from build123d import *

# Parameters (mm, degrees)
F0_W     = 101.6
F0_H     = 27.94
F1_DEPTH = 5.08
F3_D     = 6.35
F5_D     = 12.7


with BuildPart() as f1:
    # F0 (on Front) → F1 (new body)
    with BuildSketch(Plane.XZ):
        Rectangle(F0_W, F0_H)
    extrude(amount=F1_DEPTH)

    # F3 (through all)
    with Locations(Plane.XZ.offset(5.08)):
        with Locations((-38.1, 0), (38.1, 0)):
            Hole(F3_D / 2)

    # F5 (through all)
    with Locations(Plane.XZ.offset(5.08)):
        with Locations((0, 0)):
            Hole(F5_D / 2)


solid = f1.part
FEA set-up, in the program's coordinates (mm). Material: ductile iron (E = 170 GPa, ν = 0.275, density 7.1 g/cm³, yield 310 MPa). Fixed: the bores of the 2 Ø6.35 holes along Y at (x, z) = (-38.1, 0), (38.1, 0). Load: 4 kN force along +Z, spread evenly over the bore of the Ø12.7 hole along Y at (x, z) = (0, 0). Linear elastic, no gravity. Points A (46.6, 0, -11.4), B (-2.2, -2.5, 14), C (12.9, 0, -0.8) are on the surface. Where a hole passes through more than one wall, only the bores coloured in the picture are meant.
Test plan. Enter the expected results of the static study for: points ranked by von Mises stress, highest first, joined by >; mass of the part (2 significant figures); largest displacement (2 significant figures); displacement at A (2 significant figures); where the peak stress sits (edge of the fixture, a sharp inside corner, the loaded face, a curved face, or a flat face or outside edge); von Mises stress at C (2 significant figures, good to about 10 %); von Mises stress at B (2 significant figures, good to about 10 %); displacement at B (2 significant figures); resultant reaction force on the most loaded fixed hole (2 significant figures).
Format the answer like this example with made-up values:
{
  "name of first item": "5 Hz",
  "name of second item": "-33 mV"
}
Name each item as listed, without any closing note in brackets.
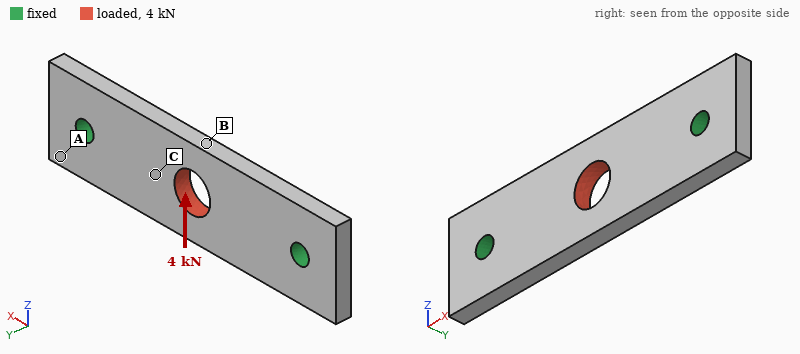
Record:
{
  "points ranked by von Mises stress, highest first, joined by >": "B > C > A",
  "mass of the part": "96 g",
  "largest displacement": "22 µm",
  "displacement at A": "5.6 µm",
  "where the peak stress sits": "edge of the fixture",
  "von Mises stress at C": "34 MPa",
  "von Mises stress at B": "85 MPa",
  "displacement at B": "21 µm",
  "resultant reaction force on the most loaded fixed hole": "2.0 kN"
}
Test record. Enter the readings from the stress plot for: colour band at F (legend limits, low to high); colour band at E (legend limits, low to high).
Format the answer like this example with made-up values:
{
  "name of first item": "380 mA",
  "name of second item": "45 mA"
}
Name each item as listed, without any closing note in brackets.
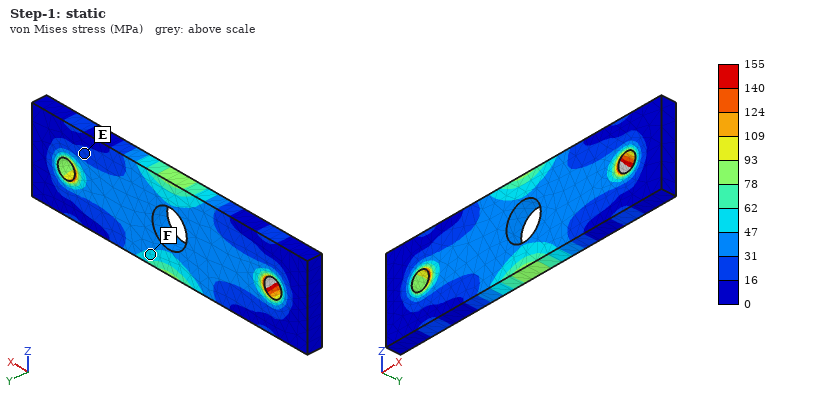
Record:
{
  "colour band at F": "47 to 62 MPa",
  "colour band at E": "16 to 31 MPa"
}
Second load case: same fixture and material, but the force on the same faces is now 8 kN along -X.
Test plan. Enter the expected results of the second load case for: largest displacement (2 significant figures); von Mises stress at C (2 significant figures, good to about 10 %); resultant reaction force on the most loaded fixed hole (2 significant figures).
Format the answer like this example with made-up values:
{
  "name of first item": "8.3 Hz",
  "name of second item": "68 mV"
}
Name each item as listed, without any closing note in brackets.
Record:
{
  "largest displacement": "7.6 µm",
  "von Mises stress at C": "39 MPa",
  "resultant reaction force on the most loaded fixed hole": "4.0 kN"
}
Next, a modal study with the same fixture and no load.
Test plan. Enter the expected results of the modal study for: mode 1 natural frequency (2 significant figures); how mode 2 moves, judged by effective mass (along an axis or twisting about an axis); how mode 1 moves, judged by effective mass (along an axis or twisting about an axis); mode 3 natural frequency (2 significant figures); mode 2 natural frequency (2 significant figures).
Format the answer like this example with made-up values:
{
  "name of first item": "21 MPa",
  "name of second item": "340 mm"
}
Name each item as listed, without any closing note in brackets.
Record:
{
  "mode 1 natural frequency": "4400 Hz",
  "how mode 2 moves, judged by effective mass": "twisting about X",
  "how mode 1 moves, judged by effective mass": "along Y",
  "mode 3 natural frequency": "11 kHz",
  "mode 2 natural frequency": "7200 Hz"
}
